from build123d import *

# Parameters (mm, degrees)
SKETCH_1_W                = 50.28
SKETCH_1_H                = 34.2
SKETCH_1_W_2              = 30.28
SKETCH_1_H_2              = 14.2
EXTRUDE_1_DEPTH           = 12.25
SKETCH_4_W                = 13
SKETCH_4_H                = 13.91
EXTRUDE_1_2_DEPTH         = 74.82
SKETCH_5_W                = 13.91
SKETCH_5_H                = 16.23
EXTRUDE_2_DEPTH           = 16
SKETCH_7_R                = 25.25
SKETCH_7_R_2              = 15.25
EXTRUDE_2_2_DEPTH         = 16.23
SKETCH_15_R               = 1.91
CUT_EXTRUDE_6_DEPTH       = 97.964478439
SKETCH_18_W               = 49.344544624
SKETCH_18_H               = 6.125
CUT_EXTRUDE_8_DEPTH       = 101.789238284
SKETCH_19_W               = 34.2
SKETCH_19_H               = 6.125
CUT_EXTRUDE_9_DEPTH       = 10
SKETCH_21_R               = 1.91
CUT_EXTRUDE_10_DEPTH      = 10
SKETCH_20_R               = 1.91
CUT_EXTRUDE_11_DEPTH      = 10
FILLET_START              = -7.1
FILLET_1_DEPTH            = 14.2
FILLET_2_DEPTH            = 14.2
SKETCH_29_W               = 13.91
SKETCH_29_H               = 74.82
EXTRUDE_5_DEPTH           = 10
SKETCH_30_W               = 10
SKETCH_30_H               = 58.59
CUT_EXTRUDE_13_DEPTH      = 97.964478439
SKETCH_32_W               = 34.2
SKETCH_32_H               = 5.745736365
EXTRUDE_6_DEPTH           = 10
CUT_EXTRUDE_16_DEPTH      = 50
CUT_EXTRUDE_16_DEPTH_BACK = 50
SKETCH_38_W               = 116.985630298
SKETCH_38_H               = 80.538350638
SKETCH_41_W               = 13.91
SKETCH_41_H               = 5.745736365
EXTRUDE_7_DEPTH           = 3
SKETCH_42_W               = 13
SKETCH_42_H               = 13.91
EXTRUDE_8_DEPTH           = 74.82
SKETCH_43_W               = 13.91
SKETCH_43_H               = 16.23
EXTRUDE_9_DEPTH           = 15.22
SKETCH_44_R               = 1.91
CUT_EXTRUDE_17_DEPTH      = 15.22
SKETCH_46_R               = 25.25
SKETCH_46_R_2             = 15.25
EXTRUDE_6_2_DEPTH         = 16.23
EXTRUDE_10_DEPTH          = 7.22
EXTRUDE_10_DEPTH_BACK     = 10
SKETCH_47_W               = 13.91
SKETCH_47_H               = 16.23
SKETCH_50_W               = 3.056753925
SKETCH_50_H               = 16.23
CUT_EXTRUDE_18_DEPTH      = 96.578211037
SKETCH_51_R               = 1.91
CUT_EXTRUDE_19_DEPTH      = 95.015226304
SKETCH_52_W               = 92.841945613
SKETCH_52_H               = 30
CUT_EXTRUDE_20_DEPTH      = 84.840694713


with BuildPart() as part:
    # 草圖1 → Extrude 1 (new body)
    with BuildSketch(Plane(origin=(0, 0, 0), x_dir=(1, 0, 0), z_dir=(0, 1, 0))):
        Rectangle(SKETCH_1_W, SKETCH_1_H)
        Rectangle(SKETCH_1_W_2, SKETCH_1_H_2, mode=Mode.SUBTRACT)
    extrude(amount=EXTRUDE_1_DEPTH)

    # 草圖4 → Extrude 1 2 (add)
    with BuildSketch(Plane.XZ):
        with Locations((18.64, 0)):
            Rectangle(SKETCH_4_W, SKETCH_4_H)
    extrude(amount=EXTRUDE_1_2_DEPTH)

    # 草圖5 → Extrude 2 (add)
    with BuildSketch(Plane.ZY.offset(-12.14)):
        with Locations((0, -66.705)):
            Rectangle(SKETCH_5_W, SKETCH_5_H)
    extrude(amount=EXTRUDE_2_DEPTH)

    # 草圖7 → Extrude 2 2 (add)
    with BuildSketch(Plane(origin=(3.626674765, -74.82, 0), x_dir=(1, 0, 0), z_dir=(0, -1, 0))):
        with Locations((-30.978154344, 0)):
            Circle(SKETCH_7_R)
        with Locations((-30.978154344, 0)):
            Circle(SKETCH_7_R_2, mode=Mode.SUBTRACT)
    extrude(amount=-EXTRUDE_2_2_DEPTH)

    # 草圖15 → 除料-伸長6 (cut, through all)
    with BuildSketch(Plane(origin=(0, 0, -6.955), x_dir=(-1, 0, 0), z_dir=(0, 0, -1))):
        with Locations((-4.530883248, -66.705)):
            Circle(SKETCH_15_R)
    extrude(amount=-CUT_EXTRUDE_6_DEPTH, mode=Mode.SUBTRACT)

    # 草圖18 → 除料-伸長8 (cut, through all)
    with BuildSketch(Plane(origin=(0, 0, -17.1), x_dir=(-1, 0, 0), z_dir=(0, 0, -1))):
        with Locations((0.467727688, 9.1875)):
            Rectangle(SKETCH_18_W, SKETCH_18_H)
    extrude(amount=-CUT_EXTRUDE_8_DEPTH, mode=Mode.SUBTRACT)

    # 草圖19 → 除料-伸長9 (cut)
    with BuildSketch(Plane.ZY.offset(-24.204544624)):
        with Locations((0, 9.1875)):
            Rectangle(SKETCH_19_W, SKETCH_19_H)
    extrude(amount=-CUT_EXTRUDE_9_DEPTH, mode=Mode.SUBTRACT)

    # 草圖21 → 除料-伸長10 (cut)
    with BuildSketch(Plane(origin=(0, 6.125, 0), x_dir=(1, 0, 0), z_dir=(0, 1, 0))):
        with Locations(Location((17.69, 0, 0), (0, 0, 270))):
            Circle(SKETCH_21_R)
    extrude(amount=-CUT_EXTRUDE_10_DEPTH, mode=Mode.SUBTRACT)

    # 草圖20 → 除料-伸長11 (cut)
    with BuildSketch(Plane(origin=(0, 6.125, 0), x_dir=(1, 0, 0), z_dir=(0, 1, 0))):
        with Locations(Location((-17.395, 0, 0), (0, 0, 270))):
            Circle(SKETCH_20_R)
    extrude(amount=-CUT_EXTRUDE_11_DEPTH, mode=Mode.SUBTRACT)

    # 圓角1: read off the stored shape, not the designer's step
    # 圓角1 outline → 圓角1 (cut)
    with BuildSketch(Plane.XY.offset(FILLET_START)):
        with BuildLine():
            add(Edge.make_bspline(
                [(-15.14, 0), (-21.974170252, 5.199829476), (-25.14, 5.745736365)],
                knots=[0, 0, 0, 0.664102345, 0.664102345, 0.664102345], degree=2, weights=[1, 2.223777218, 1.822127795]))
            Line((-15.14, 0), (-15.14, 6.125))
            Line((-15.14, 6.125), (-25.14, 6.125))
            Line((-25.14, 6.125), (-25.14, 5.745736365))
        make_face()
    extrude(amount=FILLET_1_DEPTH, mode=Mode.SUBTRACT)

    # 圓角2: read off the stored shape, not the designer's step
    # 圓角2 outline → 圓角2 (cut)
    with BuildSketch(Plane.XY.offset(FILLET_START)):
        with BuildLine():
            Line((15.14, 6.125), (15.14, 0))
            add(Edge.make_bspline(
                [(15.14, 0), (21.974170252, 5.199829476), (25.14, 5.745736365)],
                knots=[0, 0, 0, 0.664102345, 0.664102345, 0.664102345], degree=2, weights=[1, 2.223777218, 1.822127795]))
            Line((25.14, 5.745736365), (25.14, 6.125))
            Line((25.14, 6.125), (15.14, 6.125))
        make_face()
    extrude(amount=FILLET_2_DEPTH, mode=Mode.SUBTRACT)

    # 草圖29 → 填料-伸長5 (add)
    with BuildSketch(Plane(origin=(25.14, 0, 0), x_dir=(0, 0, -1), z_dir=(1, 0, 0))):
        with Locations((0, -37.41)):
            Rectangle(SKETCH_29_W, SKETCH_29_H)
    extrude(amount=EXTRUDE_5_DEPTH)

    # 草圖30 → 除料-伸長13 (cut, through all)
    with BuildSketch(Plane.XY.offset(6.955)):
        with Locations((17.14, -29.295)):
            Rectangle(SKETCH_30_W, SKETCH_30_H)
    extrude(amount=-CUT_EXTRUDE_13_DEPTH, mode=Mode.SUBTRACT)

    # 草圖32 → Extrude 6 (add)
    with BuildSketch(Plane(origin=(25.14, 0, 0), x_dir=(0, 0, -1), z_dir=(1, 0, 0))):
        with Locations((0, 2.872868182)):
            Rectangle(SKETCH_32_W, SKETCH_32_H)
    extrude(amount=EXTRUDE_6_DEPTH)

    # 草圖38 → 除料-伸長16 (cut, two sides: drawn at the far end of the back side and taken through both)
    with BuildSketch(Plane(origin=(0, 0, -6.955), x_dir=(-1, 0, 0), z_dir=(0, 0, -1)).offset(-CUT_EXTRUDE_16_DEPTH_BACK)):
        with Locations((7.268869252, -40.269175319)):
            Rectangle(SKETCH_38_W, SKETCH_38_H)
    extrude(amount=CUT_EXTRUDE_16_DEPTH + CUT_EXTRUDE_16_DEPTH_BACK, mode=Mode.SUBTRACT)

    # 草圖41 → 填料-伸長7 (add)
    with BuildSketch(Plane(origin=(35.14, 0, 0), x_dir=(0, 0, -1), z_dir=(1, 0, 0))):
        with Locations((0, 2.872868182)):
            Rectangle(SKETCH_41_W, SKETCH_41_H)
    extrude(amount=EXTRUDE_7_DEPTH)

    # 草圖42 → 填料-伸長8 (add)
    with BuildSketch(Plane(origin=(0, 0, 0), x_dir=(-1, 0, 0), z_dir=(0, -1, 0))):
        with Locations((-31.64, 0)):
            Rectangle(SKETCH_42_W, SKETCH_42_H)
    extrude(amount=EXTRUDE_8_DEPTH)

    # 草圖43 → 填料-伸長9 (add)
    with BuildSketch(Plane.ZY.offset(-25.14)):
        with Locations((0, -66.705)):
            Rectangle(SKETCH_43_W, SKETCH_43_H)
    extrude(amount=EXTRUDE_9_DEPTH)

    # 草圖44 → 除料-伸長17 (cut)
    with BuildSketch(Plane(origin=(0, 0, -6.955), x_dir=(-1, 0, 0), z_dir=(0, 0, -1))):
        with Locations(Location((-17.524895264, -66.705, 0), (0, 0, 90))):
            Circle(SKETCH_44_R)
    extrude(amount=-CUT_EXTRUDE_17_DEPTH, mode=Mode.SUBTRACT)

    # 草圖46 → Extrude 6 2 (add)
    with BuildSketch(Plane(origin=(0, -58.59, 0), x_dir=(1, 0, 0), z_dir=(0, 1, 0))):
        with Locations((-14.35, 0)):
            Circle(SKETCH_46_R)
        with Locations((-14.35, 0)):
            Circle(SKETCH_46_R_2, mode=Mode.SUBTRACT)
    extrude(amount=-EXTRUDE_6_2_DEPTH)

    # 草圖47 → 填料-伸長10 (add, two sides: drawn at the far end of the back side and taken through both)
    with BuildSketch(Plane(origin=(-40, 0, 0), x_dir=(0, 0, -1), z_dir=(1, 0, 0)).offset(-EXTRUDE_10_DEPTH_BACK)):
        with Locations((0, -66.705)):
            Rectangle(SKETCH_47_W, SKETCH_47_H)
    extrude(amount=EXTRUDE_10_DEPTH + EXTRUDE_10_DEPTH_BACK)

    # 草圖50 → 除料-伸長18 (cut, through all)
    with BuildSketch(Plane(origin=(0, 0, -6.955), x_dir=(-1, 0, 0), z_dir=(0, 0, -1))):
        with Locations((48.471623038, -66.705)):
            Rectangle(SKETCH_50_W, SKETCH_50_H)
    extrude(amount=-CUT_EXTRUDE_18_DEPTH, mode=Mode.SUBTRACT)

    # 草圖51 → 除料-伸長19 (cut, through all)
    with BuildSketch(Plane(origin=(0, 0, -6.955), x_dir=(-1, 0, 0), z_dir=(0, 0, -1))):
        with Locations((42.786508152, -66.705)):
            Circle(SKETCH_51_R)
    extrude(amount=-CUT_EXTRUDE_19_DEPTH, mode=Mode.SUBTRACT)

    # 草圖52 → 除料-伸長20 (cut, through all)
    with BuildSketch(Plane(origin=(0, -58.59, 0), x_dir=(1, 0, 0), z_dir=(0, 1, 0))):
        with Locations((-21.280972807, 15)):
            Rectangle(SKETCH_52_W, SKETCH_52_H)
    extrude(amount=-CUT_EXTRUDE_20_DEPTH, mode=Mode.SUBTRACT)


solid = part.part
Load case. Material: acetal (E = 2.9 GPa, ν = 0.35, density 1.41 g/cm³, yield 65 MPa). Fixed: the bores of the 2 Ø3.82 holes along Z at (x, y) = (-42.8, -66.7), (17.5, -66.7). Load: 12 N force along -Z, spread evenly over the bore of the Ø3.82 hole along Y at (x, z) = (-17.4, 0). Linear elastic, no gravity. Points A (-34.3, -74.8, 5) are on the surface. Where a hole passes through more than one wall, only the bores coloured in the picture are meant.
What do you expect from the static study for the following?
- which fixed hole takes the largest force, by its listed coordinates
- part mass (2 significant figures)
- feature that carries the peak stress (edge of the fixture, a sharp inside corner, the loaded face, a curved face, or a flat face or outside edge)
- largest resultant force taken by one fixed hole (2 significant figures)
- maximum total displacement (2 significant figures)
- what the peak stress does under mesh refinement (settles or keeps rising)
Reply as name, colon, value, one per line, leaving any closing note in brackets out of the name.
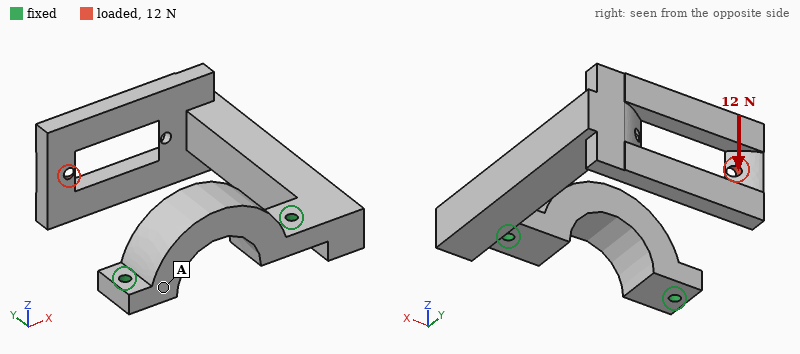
which fixed hole takes the largest force, by its listed coordinates: (17.5, -66.7)
part mass: 50 g
feature that carries the peak stress: edge of the fixture
largest resultant force taken by one fixed hole: 11 N
maximum total displacement: 1.2 mm
what the peak stress does under mesh refinement: keeps rising
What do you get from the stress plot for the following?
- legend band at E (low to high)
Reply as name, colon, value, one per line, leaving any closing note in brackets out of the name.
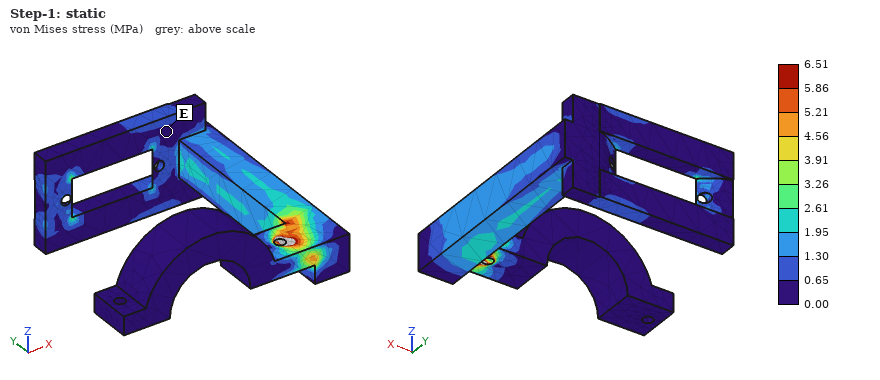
legend band at E: 0.00 to 0.65 MPa
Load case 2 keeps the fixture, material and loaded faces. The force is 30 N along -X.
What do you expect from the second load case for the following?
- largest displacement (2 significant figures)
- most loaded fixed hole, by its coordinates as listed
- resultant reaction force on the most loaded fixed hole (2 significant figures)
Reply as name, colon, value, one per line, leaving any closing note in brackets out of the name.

largest displacement: 1.2 mm
most loaded fixed hole, by its coordinates as listed: (17.5, -66.7)
resultant reaction force on the most loaded fixed hole: 35 N
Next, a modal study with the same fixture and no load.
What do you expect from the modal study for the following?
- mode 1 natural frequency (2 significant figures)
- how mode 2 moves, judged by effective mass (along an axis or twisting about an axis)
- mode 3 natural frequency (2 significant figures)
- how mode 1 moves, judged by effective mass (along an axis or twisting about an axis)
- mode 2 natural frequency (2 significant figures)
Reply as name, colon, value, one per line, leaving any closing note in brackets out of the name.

mode 1 natural frequency: 170 Hz
how mode 2 moves, judged by effective mass: along X
mode 3 natural frequency: 370 Hz
how mode 1 moves, judged by effective mass: along Z
mode 2 natural frequency: 200 Hz
